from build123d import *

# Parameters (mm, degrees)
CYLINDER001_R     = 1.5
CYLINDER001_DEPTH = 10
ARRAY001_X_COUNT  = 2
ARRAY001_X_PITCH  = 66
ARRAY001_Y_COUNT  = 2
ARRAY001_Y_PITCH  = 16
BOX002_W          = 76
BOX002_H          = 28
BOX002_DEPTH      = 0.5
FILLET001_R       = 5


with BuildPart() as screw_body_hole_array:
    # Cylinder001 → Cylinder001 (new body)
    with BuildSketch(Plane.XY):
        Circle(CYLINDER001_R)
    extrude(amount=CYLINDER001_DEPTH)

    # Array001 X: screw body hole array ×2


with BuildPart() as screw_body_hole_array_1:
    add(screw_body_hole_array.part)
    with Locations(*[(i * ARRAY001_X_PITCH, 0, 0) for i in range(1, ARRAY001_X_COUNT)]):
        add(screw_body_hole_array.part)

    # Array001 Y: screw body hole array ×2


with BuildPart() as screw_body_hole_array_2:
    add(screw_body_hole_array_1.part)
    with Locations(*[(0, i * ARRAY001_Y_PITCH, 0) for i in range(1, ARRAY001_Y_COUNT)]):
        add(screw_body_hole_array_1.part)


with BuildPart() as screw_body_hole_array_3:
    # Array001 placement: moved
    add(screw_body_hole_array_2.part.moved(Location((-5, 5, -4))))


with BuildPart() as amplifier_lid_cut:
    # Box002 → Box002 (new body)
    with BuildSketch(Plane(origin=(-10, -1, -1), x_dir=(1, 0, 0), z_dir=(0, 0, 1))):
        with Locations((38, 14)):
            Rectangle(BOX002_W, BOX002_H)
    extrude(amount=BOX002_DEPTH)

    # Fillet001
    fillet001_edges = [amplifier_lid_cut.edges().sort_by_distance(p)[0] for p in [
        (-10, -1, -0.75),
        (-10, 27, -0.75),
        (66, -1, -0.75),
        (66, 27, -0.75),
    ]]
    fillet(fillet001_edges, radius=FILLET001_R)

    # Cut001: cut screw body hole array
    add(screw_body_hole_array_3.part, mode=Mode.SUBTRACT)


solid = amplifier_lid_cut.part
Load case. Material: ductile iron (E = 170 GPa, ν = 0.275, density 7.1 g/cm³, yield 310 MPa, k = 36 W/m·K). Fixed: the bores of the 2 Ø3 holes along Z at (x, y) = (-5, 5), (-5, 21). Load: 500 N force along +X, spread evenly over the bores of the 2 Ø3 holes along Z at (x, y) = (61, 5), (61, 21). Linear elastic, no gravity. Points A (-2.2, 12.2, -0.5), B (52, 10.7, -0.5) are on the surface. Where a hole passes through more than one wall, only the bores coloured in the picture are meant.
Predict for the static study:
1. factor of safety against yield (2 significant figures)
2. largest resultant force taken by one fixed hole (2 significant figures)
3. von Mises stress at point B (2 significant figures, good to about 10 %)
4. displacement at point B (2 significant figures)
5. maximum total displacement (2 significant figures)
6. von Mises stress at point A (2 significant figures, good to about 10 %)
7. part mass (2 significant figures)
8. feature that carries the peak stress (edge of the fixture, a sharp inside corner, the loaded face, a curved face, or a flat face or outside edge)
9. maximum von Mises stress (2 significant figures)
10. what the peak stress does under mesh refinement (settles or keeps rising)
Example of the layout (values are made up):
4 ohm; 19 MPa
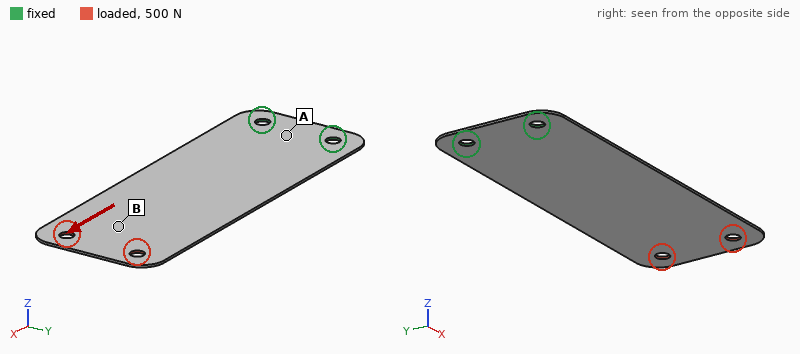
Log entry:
2.5; 250 N; 33 MPa; 12 µm; 16 µm; 17 MPa; 7.4 g; the loaded face; 130 MPa; settles
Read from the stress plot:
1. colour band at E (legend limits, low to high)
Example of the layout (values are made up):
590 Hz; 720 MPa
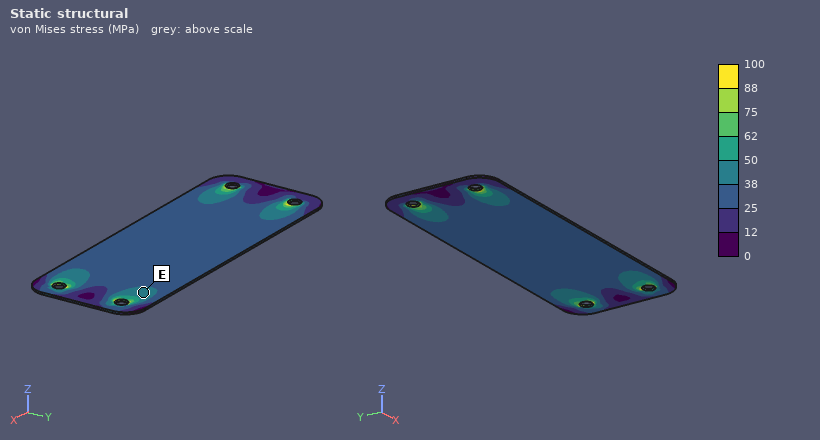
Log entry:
38 to 50 MPa
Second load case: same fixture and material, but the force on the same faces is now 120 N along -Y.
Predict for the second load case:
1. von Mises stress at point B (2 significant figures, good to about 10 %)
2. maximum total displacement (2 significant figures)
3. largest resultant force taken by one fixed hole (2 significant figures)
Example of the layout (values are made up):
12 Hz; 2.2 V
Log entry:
22 MPa; 0.11 mm; 450 N
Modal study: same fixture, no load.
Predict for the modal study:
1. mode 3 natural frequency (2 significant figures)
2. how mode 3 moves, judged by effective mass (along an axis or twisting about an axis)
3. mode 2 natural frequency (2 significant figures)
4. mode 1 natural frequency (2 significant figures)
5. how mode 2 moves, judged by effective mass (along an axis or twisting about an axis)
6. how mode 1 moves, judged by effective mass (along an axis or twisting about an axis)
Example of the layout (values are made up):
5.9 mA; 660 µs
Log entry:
510 Hz; along Z; 440 Hz; 82 Hz; twisting about X; along Z
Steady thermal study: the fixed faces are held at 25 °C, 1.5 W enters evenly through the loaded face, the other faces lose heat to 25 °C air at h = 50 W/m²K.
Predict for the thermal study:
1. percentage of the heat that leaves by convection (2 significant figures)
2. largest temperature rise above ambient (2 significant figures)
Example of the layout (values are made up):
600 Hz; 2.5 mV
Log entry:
99 %; 36 K
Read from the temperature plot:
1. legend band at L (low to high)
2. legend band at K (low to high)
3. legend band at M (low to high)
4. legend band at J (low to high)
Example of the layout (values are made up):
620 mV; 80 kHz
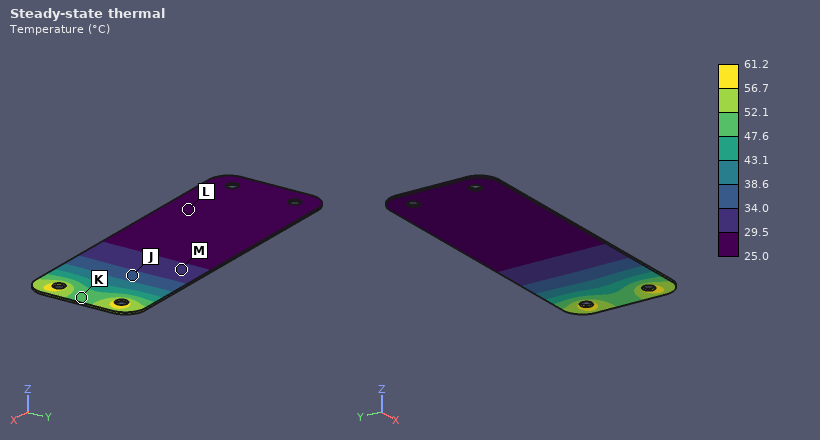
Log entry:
25.0 to 29.5 °C; 47.6 to 52.1 °C; 29.5 to 34.0 °C; 34.0 to 38.6 °C
